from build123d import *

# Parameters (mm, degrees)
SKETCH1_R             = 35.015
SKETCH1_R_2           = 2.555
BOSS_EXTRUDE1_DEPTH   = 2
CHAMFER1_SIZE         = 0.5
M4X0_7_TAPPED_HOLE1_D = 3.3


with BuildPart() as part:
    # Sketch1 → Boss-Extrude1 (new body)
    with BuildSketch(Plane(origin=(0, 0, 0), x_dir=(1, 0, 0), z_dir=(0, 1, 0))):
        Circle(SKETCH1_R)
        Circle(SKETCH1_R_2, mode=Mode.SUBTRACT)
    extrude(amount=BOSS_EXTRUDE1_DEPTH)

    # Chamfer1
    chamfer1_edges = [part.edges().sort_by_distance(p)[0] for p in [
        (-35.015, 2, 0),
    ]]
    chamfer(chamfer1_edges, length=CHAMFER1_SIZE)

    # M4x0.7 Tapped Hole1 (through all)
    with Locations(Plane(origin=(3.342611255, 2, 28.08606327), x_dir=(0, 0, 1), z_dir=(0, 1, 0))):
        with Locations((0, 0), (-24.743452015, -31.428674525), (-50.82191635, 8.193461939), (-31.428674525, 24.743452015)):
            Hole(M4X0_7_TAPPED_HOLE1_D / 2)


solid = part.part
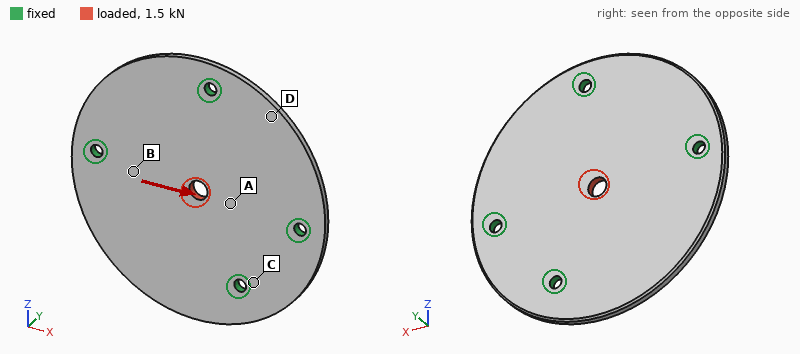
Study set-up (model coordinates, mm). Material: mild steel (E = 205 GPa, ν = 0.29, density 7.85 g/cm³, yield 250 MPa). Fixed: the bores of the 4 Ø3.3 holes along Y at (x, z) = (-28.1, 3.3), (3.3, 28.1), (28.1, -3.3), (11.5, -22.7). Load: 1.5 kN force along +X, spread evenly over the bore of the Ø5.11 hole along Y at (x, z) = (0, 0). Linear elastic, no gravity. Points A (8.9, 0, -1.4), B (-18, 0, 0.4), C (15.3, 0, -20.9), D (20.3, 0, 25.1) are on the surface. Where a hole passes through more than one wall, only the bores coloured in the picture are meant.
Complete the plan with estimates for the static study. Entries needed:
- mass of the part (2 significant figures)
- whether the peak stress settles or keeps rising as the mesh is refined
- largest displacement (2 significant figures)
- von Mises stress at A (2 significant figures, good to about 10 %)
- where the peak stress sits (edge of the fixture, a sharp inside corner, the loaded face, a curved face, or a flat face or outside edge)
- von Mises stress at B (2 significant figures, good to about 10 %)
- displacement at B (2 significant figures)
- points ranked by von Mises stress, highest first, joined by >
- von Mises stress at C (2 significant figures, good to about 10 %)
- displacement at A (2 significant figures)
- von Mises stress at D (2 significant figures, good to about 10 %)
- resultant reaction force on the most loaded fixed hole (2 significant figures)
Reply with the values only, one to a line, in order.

59 g
keeps rising
3.0 µm
25 MPa
a sharp inside corner
19 MPa
1.0 µm
A > B > C > D
10 MPa
1.8 µm
5.5 MPa
460 N
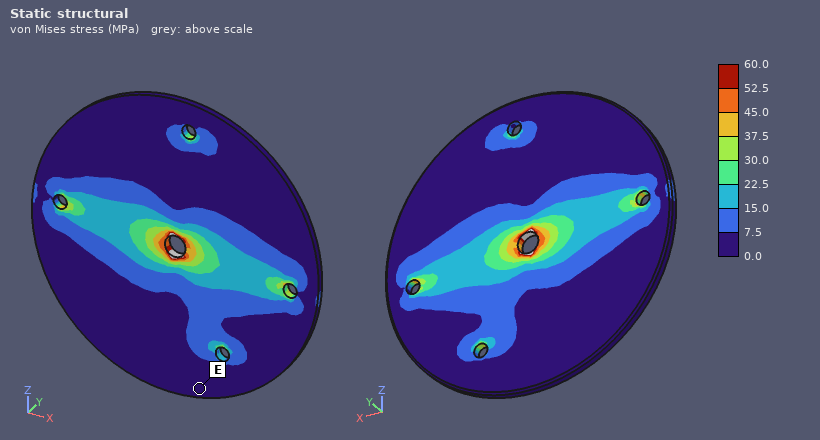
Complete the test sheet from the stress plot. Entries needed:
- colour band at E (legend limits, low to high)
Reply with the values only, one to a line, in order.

0.0 to 7.5 MPa
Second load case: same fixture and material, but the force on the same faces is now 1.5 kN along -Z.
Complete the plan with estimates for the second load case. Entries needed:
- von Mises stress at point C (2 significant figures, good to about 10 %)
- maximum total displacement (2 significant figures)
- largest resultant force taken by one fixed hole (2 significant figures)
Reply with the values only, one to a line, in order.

7.4 MPa
3.2 µm
490 N
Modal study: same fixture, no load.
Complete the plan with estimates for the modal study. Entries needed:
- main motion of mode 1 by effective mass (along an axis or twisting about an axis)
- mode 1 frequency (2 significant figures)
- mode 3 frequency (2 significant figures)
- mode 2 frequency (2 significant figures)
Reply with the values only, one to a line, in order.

along Y
2900 Hz
5100 Hz
5000 Hz
